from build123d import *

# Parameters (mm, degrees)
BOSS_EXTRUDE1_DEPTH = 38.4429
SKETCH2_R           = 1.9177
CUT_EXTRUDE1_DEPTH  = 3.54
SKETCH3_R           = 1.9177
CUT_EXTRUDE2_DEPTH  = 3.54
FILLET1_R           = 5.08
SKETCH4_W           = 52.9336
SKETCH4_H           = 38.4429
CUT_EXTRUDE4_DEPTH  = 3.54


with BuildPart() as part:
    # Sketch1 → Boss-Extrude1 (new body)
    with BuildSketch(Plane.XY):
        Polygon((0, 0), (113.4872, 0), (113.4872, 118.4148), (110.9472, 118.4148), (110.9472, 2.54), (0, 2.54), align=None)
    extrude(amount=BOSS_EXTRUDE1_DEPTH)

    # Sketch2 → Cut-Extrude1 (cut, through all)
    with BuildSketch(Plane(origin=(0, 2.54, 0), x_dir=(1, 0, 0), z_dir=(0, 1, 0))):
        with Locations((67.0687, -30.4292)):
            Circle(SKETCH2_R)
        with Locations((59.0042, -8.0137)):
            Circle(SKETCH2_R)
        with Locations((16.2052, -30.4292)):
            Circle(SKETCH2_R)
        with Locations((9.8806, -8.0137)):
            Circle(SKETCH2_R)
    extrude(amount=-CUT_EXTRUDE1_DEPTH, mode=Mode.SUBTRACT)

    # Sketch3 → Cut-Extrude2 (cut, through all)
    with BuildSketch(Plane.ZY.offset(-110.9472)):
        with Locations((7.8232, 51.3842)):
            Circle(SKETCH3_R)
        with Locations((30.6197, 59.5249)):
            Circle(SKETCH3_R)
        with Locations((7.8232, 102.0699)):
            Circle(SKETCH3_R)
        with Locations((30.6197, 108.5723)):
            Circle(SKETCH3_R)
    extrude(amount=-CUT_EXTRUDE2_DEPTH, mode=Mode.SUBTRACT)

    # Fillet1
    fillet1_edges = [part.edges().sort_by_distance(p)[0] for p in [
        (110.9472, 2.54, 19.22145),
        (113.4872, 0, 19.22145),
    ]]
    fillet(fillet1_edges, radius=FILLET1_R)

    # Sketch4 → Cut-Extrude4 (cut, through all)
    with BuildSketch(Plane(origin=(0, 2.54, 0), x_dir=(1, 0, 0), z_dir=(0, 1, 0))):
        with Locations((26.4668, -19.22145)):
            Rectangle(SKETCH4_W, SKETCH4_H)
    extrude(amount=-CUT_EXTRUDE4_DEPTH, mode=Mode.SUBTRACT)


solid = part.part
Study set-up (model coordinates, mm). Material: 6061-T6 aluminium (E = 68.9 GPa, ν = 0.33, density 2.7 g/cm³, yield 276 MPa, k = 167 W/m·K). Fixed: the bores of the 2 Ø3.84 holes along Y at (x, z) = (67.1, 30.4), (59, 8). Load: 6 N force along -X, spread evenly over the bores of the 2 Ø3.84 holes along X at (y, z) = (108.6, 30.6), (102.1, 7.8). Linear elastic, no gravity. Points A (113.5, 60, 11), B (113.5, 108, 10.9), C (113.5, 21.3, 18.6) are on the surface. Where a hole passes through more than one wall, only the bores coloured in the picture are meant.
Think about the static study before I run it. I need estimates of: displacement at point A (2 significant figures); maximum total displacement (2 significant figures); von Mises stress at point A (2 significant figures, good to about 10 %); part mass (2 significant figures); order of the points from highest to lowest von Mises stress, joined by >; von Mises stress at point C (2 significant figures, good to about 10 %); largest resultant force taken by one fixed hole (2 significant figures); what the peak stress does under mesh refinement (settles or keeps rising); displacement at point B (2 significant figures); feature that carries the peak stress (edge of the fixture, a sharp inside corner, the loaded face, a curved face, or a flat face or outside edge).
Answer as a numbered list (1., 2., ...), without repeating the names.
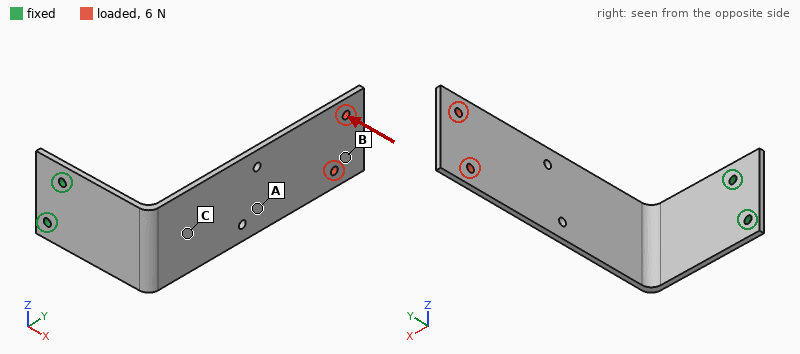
1. 0.66 mm
2. 1.5 mm
3. 6.6 MPa
4. 46 g
5. C > A > B
6. 11 MPa
7. 9.0 N
8. keeps rising
9. 1.4 mm
10. edge of the fixture
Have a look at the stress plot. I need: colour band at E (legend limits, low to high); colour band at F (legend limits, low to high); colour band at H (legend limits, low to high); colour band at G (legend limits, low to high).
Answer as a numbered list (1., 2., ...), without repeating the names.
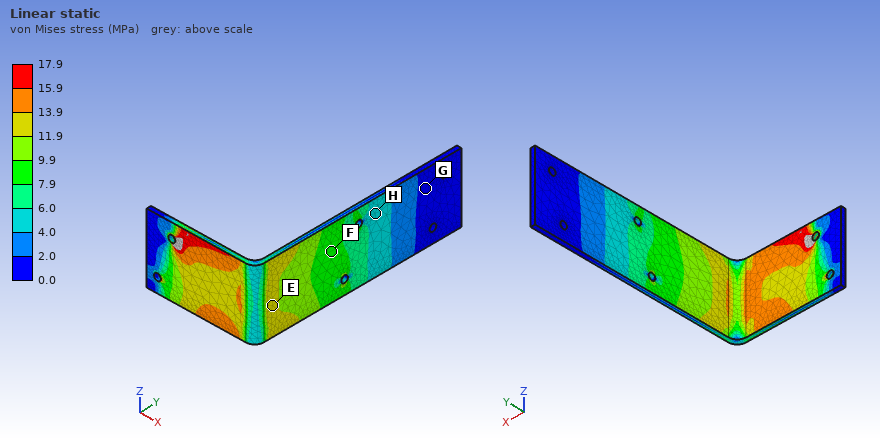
1. 11.9 to 13.9 MPa
2. 7.9 to 9.9 MPa
3. 4.0 to 6.0 MPa
4. 0.0 to 2.0 MPa
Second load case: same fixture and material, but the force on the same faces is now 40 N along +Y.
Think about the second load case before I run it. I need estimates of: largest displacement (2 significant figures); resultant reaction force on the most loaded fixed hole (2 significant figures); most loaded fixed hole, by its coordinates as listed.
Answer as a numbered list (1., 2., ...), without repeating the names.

1. 1.5 mm
2. 45 N
3. (67.1, 30.4)
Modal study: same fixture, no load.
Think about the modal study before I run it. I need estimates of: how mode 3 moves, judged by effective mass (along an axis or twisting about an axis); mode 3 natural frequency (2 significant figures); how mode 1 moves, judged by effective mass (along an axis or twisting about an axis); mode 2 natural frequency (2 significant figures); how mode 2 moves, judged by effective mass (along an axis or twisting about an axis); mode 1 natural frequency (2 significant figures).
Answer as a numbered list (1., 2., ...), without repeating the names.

1. along Y
2. 390 Hz
3. along X
4. 170 Hz
5. along Z
6. 97 Hz
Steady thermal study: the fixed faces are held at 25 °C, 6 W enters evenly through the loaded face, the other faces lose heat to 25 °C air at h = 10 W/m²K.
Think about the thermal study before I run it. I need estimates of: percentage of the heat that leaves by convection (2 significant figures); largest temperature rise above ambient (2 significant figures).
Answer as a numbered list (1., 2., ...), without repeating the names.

1. 43 %
2. 40 K
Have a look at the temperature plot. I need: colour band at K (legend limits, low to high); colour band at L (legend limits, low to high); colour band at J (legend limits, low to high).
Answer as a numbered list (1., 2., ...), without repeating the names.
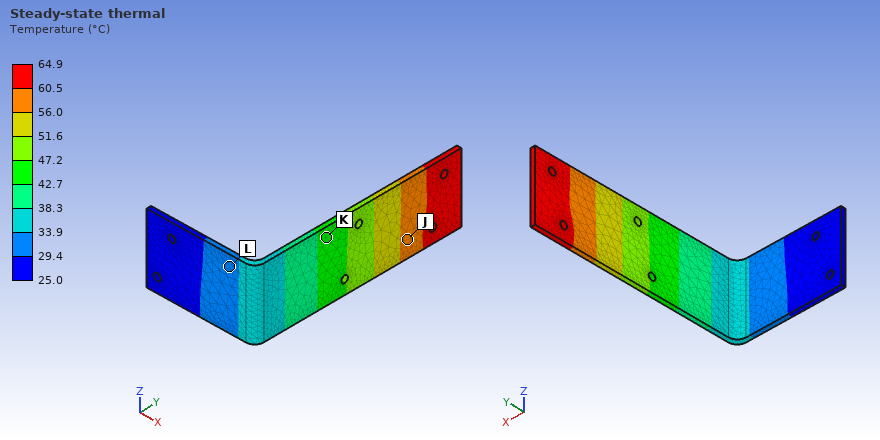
1. 42.7 to 47.2 °C
2. 29.4 to 33.9 °C
3. 56.0 to 60.5 °C
